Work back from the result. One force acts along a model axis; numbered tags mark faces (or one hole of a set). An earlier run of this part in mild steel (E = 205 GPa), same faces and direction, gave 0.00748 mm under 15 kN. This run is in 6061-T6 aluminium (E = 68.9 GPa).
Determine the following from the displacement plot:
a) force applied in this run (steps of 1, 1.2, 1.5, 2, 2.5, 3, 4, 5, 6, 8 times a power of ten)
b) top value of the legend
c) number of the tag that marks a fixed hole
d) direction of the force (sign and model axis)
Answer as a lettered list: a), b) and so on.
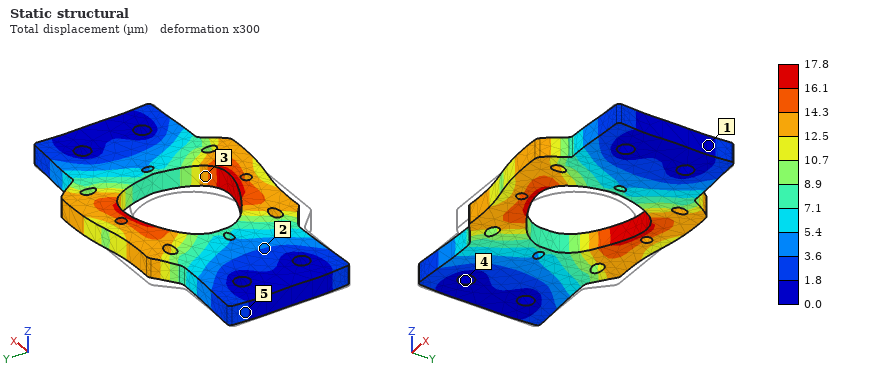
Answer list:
a) 12 kN
b) 17.8 µm
c) 4
d) +X
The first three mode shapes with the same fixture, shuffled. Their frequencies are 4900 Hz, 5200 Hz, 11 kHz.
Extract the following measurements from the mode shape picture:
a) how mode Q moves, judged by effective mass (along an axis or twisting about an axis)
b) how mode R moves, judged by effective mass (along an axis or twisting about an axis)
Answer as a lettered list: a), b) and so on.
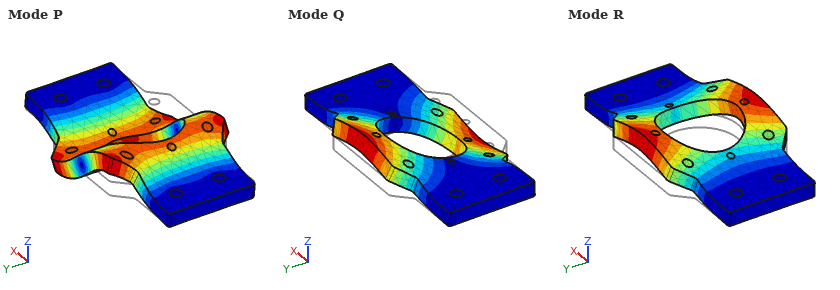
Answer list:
a) twisting about X
b) along Z
